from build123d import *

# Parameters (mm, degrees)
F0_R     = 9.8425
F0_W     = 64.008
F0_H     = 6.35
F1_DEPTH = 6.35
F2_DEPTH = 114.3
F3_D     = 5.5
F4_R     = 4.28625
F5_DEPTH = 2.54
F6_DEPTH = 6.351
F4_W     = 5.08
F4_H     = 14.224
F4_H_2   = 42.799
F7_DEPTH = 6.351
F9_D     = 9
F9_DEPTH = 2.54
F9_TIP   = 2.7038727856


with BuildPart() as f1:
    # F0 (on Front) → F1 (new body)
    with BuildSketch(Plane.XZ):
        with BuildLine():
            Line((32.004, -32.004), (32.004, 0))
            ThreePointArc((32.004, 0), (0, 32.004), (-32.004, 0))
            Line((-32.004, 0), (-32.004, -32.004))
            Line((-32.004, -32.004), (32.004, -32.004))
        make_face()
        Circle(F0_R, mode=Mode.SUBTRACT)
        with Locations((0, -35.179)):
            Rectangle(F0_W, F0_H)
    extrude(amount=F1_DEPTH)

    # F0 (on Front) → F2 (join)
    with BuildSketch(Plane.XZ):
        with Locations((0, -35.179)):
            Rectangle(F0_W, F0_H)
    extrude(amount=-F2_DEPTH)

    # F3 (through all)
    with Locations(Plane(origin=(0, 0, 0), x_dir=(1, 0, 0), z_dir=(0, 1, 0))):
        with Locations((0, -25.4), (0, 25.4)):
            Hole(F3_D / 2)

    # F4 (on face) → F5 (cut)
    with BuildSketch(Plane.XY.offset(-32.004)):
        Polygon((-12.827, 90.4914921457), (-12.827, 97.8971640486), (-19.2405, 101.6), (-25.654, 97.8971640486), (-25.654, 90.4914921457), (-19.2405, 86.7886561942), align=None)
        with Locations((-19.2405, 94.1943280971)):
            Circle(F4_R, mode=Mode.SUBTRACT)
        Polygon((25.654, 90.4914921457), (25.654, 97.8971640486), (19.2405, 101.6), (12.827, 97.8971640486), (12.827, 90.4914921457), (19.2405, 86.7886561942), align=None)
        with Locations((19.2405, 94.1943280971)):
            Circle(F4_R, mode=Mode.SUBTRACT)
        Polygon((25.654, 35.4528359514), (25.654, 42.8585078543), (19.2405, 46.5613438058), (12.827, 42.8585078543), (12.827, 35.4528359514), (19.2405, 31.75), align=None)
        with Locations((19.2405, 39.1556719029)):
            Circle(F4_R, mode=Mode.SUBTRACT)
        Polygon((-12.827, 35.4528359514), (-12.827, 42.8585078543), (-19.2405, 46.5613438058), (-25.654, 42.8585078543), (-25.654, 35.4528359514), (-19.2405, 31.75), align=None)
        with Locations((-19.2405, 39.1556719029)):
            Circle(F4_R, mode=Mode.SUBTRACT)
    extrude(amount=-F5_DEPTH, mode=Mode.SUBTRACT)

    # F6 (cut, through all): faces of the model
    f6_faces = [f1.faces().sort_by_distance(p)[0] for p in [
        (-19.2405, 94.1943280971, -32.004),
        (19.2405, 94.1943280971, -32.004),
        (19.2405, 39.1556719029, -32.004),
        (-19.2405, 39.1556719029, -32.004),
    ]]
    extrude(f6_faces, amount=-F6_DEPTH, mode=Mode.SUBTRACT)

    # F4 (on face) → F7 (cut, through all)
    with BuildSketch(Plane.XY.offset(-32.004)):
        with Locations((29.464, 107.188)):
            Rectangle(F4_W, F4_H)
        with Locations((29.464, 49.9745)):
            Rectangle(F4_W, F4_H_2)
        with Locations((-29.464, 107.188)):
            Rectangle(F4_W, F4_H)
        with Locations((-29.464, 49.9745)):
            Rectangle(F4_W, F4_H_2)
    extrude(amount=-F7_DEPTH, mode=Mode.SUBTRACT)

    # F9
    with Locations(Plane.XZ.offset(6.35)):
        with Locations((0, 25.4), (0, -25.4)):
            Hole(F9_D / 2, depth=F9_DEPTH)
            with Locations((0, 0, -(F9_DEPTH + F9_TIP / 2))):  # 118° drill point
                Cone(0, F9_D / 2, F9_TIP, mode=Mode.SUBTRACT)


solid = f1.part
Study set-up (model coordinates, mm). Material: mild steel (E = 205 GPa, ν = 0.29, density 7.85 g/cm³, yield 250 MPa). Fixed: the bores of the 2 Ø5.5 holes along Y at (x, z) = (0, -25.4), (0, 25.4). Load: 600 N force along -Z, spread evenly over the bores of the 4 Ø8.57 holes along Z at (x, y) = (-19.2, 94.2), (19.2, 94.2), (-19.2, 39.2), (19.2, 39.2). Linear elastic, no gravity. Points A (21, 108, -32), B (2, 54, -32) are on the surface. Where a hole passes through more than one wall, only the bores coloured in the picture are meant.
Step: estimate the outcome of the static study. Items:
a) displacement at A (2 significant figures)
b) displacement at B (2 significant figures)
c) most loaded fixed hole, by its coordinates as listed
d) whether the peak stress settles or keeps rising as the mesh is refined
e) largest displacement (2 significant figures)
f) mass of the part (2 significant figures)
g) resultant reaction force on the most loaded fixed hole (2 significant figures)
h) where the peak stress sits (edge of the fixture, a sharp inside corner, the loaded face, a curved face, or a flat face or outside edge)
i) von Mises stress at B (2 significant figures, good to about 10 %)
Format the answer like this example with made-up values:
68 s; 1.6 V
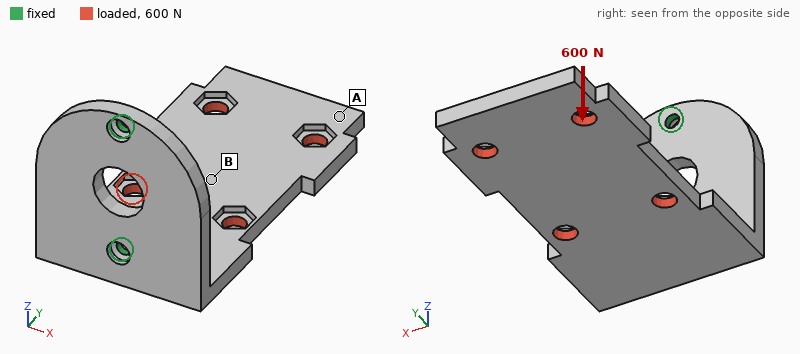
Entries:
0.85 mm; 0.34 mm; (0, -25.4); keeps rising; 0.92 mm; 500 g; 1.8 kN; edge of the fixture; 39 MPa
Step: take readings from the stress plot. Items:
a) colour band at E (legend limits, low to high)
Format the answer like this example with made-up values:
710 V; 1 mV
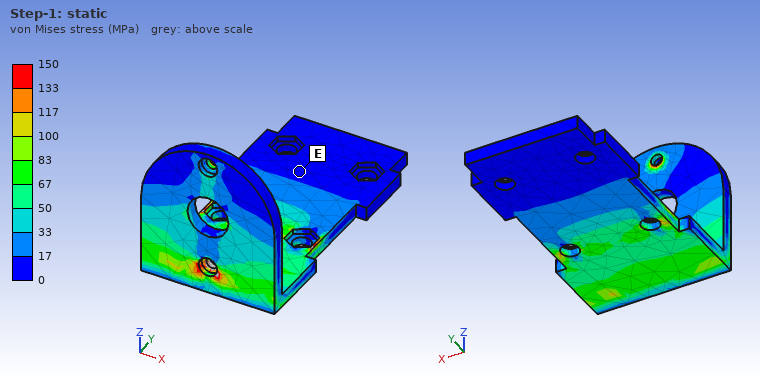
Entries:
0 to 17 MPa
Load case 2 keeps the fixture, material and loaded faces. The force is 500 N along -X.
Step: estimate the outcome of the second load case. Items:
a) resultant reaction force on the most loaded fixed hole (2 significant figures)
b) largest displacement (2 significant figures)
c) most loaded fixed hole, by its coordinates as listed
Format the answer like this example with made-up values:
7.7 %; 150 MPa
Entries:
630 N; 0.34 mm; (0, -25.4)
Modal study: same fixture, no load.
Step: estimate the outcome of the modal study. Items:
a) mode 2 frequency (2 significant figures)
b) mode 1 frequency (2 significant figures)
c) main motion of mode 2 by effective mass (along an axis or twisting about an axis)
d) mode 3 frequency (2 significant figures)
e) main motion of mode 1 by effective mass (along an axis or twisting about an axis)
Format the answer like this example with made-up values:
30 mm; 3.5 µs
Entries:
440 Hz; 310 Hz; along X; 1500 Hz; along Z
